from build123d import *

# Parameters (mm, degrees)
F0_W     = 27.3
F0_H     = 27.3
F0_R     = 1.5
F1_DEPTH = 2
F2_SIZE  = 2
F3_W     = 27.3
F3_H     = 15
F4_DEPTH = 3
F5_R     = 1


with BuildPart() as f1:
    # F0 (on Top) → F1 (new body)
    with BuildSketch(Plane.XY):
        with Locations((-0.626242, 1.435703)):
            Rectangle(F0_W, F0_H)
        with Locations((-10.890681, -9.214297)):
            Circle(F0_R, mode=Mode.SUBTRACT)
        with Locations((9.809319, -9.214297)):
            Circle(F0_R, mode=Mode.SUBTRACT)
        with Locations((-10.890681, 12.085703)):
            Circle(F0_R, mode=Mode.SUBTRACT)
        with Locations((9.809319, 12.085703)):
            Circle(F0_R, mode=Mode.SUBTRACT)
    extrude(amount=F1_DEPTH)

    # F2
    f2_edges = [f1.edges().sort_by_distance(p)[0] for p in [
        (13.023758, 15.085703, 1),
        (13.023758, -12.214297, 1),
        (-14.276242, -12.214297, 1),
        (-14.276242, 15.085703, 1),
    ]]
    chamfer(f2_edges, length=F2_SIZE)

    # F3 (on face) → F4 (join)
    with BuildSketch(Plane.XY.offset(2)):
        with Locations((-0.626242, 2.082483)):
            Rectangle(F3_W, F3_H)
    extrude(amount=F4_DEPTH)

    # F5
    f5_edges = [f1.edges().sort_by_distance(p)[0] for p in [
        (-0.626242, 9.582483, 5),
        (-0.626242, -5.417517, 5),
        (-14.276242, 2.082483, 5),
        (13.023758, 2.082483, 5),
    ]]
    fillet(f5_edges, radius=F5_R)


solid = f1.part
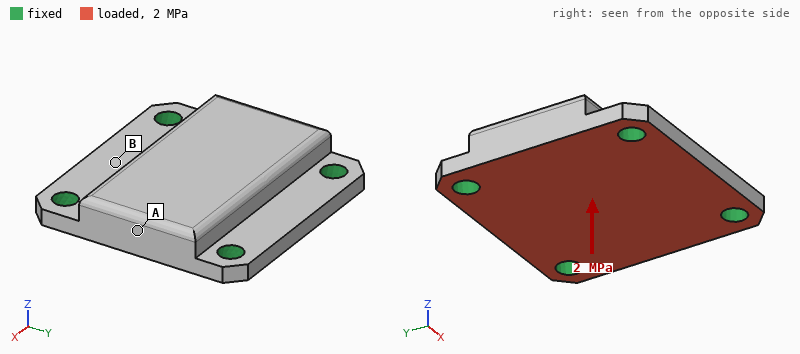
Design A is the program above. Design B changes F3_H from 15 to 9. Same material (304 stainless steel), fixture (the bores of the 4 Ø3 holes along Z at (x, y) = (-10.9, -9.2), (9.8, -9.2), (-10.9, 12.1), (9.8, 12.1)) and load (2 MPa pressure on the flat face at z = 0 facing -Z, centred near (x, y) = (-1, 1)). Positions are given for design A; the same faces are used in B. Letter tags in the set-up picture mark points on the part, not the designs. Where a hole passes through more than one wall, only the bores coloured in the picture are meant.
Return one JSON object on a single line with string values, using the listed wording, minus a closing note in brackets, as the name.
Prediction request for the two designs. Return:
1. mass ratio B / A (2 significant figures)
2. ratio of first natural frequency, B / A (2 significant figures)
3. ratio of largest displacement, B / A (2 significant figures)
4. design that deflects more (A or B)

{"mass ratio B / A": "0.81", "ratio of first natural frequency, B / A": "0.80", "ratio of largest displacement, B / A": "1.5", "design that deflects more": "B"}
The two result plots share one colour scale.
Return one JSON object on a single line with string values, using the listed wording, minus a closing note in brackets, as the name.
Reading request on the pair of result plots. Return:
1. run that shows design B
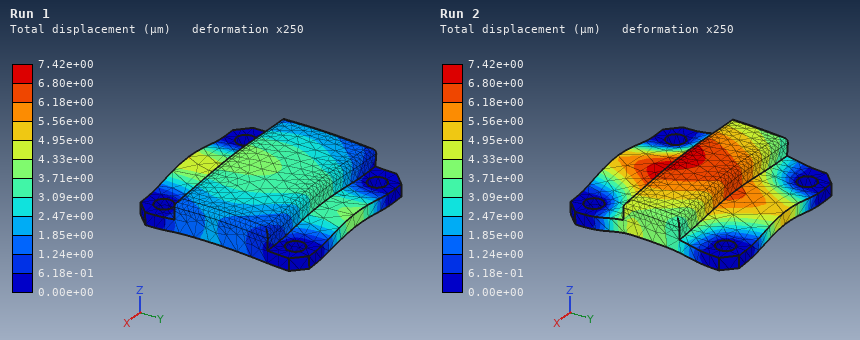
{"run that shows design B": "Run 2"}
